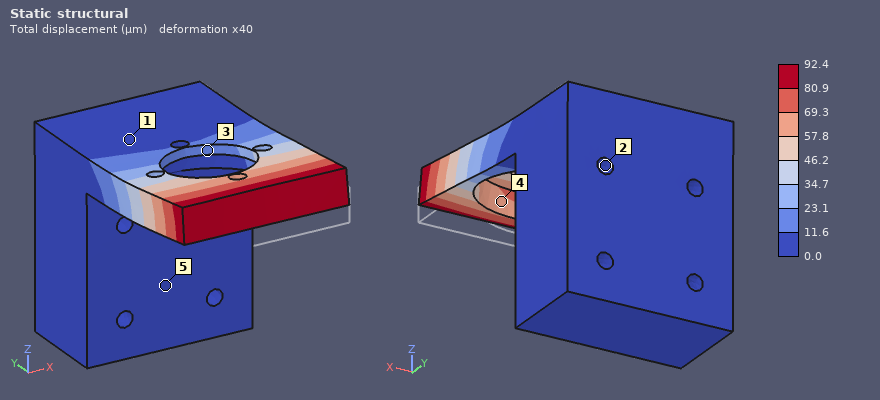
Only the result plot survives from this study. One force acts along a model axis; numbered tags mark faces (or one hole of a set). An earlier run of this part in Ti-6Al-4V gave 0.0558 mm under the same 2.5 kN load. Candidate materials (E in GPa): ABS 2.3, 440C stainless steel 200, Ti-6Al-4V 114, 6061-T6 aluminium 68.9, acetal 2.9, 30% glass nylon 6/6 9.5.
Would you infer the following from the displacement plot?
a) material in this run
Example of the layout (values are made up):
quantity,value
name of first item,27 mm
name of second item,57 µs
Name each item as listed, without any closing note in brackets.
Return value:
quantity,value
material in this run,6061-T6 aluminium
